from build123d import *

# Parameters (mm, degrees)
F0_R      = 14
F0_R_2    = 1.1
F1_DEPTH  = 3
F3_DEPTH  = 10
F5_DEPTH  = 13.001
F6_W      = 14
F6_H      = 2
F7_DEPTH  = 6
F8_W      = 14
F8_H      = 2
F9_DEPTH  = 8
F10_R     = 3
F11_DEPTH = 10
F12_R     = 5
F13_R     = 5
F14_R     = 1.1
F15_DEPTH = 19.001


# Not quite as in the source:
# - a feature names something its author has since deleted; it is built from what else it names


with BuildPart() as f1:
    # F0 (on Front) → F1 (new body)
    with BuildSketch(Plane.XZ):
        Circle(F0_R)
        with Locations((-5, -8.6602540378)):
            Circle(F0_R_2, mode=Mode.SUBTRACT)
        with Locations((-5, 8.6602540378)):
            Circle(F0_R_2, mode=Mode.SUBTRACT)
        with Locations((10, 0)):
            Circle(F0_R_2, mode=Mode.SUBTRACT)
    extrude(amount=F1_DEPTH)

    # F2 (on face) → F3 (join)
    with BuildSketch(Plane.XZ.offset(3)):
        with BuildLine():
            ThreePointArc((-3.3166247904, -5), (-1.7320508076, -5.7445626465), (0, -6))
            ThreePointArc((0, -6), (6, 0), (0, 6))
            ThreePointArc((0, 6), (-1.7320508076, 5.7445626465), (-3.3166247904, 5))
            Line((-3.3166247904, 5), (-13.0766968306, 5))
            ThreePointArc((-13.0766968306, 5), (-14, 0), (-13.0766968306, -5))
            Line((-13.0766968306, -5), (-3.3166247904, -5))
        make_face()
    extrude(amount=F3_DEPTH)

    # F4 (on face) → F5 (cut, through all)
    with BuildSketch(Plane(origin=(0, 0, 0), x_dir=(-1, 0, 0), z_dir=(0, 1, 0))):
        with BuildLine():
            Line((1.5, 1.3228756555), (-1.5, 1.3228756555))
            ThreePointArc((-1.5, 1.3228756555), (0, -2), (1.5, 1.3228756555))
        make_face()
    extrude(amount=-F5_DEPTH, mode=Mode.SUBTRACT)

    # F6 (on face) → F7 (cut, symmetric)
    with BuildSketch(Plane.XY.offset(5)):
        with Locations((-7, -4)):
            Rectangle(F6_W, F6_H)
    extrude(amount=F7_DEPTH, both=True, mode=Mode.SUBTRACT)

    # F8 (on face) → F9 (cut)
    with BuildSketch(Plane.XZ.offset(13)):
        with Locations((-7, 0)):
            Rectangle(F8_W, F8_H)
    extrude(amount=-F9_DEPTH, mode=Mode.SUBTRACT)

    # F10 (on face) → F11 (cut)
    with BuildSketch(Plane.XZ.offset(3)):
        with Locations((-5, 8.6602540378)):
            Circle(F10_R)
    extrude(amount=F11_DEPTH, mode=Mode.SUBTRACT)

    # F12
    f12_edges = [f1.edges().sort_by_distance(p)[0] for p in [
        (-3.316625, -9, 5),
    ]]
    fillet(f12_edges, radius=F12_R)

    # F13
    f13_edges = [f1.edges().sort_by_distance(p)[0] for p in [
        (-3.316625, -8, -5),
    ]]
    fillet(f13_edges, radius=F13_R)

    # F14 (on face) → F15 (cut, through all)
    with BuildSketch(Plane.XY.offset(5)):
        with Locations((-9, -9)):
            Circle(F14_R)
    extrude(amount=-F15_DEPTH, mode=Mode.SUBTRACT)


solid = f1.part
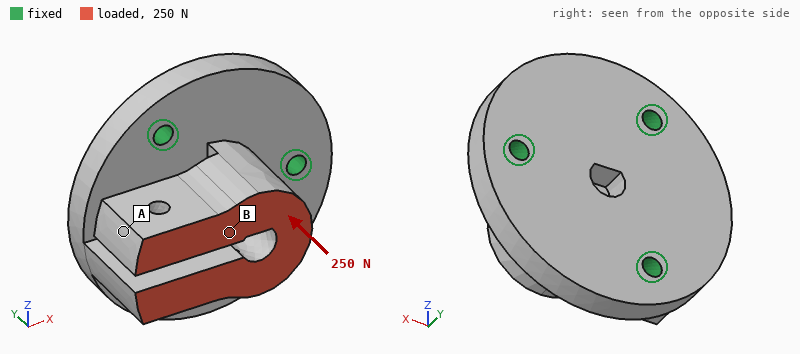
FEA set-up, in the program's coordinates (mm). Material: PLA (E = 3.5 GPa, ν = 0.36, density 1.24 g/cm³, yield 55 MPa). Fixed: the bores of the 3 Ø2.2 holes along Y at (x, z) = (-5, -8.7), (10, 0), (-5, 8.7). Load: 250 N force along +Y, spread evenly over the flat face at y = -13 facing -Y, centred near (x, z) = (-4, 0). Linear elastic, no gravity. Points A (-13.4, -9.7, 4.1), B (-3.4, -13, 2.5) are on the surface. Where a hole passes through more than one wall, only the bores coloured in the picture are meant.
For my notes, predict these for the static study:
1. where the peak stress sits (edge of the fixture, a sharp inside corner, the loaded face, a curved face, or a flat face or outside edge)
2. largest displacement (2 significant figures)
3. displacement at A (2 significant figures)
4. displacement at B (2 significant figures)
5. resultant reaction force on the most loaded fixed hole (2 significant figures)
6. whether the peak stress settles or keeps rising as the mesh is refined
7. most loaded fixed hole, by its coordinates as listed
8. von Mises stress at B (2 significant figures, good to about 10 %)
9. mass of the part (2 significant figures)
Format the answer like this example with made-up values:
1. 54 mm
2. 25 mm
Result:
1. edge of the fixture
2. 0.38 mm
3. 0.35 mm
4. 0.19 mm
5. 120 N
6. keeps rising
7. (-5, -8.7)
8. 8.8 MPa
9. 4.0 g
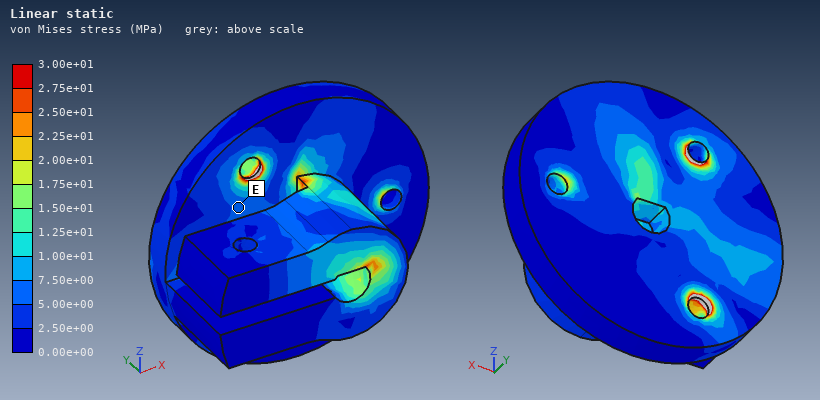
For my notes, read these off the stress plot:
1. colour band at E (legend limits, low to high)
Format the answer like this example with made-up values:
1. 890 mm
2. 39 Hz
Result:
1. 5.00e+00 to 7.50e+00 MPa
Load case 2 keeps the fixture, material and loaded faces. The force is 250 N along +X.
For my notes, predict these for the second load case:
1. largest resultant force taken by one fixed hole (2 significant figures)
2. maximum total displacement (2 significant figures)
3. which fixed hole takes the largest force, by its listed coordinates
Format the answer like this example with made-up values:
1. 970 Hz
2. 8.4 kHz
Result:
1. 220 N
2. 0.49 mm
3. (10, 0)
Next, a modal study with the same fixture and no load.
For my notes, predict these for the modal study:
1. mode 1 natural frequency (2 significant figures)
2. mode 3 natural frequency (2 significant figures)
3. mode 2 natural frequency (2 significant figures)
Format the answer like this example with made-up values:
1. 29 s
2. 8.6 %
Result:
1. 3100 Hz
2. 6600 Hz
3. 4000 Hz
